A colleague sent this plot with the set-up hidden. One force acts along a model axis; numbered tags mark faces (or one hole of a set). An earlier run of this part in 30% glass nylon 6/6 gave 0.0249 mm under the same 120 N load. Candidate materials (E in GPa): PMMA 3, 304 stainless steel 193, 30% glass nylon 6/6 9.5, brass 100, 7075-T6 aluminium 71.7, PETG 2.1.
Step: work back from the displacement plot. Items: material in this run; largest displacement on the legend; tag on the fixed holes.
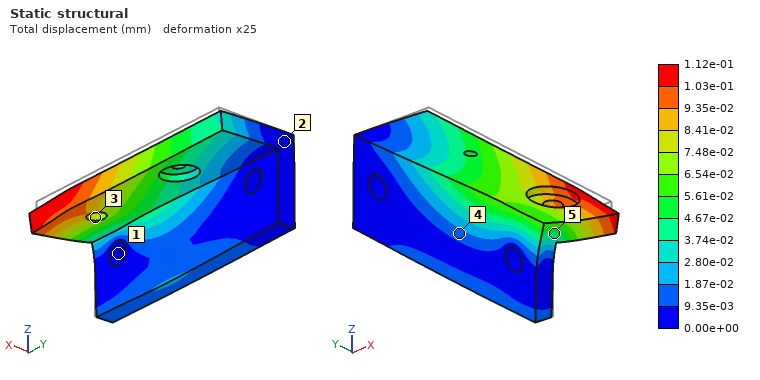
PETG
1.12e-01 mm
1
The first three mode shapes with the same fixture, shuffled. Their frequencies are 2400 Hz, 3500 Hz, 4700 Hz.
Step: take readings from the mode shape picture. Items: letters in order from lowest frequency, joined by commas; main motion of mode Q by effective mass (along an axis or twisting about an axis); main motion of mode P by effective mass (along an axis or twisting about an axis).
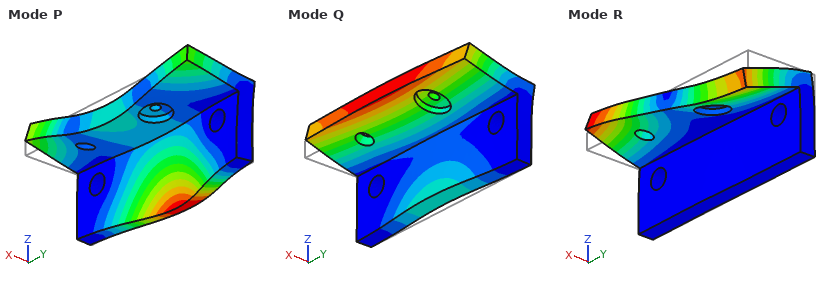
Q, R, P
along Z
along X
